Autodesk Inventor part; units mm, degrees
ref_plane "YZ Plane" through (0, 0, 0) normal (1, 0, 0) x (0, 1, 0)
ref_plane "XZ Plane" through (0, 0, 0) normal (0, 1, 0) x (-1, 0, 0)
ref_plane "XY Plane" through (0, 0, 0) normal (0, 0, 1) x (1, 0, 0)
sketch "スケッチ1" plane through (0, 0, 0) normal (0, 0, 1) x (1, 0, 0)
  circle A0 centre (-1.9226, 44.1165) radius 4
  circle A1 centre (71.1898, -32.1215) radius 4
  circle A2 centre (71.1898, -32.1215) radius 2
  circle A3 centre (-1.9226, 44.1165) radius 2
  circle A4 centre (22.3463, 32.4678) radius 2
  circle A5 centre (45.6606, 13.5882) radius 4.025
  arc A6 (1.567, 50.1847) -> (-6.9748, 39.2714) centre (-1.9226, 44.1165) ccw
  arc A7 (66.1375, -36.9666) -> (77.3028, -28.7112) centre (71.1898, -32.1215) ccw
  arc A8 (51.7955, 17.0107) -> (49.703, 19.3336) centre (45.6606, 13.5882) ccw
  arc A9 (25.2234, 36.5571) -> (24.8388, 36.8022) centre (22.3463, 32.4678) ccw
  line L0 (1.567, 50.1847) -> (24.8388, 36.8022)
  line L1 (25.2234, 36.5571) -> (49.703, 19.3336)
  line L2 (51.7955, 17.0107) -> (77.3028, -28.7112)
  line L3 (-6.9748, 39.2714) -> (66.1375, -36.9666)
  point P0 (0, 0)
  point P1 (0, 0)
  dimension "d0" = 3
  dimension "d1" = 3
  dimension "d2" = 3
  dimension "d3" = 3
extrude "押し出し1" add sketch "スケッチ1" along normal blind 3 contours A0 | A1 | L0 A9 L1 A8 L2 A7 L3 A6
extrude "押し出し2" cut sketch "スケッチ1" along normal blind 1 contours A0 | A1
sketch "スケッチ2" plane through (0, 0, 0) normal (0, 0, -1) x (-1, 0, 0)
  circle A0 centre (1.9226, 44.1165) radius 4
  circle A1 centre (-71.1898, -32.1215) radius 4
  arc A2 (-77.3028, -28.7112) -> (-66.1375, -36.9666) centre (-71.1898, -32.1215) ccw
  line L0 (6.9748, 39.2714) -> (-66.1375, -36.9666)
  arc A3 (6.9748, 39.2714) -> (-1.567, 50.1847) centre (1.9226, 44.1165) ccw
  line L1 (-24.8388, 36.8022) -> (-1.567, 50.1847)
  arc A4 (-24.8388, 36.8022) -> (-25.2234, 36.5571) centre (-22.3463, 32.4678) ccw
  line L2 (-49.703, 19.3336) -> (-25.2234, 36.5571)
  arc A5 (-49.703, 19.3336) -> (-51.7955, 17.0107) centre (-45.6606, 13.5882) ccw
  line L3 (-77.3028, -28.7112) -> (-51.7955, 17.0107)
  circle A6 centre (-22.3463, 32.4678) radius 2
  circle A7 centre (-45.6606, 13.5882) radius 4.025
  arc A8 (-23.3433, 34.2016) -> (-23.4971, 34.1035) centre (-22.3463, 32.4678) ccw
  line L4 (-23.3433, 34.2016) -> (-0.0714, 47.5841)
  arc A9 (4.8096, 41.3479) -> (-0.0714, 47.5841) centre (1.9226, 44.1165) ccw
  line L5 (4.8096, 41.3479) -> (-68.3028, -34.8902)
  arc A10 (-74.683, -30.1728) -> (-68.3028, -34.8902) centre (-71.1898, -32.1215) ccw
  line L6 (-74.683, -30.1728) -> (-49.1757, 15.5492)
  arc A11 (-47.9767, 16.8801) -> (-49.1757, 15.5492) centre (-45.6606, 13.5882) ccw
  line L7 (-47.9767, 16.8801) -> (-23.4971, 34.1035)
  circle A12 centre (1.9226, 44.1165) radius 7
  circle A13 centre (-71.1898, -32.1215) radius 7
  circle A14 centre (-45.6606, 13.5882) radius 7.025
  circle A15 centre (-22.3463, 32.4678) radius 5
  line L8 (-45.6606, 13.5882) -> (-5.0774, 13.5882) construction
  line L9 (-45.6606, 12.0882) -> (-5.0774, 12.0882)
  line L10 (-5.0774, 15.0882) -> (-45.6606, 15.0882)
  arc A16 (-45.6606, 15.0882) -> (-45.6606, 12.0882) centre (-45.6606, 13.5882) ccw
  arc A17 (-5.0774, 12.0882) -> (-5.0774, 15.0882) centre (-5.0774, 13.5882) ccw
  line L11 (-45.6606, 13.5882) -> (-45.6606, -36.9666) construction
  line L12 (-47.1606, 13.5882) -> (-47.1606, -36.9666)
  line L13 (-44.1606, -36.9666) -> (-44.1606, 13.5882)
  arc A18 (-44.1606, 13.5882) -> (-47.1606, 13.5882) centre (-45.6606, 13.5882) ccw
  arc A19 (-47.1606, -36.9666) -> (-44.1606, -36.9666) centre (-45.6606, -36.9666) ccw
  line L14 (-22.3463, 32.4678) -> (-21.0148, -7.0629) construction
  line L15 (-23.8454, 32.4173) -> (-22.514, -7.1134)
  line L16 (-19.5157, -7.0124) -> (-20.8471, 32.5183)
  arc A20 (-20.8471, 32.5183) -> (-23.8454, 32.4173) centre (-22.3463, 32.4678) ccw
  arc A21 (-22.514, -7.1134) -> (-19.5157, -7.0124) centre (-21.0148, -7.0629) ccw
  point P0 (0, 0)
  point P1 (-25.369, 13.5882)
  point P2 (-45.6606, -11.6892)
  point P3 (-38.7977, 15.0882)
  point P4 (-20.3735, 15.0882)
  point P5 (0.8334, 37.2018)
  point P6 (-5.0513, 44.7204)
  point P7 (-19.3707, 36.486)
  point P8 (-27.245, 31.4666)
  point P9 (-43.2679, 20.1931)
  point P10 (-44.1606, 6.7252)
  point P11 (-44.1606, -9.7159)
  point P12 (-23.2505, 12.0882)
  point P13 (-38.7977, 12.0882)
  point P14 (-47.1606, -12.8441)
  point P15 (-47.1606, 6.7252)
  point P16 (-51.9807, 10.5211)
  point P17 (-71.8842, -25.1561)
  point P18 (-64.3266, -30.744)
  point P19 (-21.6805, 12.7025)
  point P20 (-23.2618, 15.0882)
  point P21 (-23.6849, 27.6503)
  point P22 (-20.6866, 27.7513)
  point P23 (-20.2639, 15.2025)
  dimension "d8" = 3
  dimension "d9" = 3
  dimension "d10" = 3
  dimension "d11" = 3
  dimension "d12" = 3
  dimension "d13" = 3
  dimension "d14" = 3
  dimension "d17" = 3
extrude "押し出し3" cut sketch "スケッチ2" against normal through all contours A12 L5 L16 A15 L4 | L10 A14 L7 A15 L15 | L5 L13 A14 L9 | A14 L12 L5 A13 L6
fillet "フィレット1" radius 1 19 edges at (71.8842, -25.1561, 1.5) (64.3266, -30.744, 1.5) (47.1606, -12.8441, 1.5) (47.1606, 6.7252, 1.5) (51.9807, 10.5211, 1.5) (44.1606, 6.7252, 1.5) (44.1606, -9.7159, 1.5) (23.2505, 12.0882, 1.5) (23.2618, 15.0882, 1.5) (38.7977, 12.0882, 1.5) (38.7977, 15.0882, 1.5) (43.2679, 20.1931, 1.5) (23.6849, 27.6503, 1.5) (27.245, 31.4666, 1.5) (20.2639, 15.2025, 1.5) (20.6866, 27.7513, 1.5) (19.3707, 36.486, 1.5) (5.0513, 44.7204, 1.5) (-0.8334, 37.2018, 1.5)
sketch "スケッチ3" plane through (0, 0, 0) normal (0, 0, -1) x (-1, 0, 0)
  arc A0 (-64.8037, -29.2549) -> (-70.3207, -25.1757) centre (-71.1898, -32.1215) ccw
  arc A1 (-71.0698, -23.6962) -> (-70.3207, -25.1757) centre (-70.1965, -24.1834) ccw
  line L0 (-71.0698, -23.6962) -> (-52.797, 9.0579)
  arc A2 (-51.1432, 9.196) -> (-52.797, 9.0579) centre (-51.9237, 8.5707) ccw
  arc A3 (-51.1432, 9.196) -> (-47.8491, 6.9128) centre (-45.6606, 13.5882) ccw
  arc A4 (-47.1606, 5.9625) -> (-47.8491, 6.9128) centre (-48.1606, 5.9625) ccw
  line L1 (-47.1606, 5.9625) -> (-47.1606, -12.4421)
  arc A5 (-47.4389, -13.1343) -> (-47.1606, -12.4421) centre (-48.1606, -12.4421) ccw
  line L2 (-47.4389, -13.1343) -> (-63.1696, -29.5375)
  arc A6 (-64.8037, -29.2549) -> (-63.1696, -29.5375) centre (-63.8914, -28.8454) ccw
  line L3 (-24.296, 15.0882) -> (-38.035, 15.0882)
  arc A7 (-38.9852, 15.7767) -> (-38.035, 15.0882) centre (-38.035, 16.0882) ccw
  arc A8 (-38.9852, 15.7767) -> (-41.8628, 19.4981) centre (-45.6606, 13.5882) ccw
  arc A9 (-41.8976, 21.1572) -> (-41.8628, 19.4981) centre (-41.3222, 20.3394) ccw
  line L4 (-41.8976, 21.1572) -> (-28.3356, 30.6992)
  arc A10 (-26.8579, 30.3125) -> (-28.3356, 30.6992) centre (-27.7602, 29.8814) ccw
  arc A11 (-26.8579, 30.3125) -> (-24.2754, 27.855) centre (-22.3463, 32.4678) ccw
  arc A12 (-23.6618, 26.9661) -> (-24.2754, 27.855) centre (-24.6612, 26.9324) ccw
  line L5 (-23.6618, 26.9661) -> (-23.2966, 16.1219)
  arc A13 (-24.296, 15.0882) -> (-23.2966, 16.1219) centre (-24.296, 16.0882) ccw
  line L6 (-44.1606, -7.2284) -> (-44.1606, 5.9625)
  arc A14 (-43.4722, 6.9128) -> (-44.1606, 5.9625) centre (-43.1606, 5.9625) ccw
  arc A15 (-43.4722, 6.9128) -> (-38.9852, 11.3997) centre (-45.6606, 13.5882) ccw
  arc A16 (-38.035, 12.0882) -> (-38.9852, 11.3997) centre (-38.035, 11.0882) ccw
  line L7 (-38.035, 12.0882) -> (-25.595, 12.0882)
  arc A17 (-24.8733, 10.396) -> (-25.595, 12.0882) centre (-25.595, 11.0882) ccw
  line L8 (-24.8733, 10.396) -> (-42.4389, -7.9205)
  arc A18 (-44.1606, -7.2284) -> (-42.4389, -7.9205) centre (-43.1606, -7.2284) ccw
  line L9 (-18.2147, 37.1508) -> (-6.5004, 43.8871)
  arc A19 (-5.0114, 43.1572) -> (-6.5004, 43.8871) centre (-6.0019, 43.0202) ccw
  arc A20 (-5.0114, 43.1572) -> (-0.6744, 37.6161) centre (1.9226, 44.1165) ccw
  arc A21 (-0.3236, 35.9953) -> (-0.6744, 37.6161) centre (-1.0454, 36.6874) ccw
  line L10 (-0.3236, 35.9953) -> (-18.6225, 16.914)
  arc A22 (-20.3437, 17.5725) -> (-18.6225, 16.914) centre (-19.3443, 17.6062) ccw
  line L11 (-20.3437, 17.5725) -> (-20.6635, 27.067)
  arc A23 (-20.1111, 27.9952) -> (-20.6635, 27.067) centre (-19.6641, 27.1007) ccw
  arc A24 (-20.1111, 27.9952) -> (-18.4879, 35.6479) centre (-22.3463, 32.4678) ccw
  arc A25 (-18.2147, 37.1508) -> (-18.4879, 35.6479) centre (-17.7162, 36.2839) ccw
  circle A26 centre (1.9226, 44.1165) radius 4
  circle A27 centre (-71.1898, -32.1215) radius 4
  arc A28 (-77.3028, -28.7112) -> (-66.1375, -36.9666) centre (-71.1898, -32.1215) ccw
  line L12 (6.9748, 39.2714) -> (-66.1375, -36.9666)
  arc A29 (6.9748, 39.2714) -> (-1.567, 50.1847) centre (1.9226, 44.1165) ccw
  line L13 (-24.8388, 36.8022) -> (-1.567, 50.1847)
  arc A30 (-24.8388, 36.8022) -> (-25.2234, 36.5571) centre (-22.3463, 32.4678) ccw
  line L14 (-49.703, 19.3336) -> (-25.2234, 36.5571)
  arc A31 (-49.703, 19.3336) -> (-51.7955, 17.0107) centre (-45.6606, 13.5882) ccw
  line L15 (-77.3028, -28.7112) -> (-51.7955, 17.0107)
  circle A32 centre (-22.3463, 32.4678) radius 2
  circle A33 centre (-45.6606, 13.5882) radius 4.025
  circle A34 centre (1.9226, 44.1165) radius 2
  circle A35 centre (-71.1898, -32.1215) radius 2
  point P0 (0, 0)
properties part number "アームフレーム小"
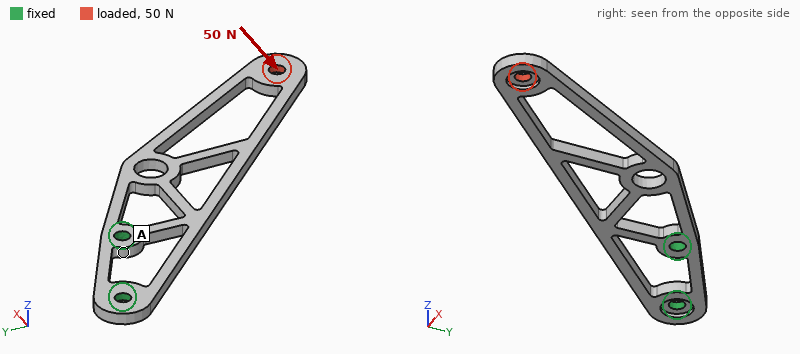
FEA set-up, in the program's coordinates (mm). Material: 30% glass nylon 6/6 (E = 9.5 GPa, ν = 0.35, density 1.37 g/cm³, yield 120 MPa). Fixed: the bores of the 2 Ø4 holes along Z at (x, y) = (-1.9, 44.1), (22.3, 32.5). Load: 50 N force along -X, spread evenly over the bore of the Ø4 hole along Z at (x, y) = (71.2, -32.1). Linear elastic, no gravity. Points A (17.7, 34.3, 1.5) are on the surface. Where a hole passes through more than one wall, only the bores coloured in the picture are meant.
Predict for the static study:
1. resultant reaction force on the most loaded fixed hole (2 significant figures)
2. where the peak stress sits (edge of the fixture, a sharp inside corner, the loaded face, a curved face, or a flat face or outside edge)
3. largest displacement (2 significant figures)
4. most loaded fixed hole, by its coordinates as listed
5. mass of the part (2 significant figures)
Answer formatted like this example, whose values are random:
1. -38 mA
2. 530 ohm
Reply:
1. 180 N
2. a curved face
3. 1.3 mm
4. (-1.9, 44.1)
5. 4.6 g
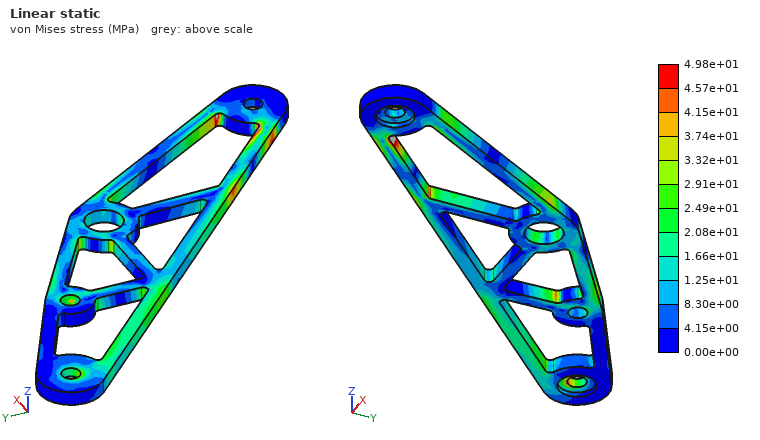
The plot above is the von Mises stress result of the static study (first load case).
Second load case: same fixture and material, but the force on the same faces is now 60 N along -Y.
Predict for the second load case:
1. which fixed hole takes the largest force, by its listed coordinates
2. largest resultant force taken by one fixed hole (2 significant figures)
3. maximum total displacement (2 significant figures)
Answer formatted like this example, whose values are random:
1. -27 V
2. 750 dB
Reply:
1. (22.3, 32.5)
2. 200 N
3. 1.3 mm
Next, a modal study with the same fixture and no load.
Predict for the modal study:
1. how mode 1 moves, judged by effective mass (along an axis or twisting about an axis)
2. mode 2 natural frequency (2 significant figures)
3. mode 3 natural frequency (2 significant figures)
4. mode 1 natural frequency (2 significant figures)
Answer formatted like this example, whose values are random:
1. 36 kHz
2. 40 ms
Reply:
1. along Z
2. 870 Hz
3. 880 Hz
4. 160 Hz
